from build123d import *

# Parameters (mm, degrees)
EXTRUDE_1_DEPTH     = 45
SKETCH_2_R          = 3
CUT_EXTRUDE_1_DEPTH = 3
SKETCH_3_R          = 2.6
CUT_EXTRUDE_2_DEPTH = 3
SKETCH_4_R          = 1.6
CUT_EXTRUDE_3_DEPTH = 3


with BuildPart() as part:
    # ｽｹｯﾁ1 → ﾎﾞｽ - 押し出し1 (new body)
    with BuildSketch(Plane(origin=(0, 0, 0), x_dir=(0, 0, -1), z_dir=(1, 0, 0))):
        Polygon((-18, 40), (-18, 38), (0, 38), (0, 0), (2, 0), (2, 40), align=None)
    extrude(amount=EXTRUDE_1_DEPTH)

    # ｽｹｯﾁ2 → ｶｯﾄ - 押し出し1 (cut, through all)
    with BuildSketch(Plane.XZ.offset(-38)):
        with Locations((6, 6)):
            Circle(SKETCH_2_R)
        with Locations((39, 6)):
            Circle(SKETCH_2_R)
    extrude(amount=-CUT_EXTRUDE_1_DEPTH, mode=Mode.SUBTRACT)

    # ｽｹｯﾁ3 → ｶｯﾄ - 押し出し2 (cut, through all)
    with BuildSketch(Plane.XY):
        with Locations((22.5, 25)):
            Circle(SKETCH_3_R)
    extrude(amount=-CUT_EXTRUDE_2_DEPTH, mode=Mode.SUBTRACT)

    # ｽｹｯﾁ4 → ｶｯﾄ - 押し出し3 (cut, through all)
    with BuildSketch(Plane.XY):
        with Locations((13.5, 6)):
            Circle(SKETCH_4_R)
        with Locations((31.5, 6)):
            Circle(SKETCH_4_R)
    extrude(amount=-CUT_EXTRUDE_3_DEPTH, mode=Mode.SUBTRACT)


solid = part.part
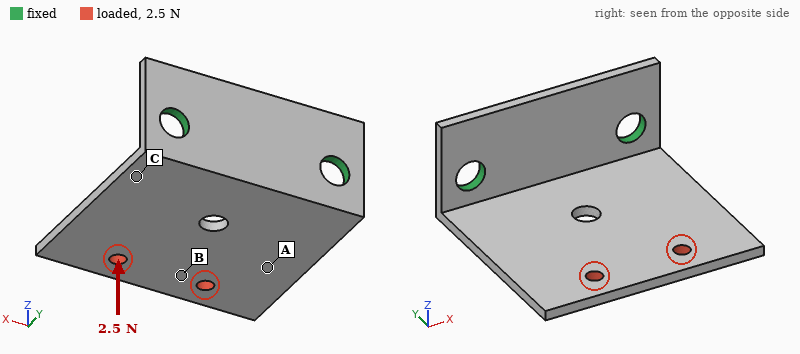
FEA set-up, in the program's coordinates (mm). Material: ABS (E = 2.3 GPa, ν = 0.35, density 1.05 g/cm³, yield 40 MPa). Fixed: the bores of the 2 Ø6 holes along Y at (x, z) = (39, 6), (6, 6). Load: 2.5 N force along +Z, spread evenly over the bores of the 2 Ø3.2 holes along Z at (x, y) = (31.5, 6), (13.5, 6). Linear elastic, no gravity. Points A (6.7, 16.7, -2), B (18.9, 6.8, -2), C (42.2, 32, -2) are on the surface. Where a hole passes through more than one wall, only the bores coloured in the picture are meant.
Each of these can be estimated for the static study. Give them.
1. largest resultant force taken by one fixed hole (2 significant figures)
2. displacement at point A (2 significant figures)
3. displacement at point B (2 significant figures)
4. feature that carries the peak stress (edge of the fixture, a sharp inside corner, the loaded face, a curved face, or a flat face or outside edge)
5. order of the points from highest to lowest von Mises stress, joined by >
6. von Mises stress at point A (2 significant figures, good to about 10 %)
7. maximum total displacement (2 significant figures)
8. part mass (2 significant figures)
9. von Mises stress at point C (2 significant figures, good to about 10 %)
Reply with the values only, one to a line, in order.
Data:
1.3 N
0.34 mm
0.59 mm
a flat face or outside edge
C > A > B
0.96 MPa
0.76 mm
5.3 g
2.2 MPa
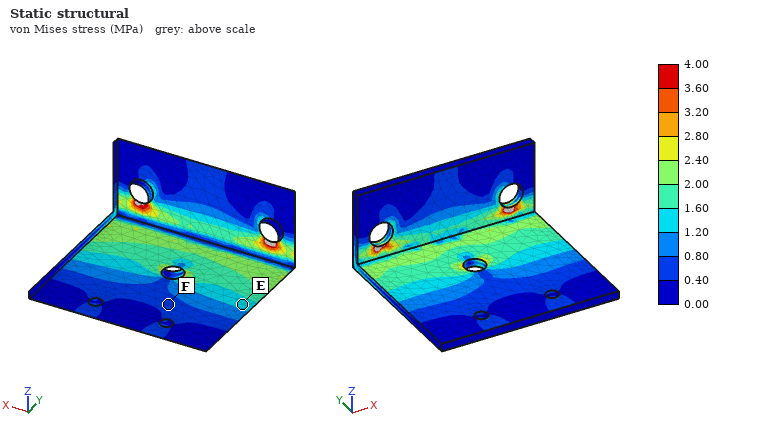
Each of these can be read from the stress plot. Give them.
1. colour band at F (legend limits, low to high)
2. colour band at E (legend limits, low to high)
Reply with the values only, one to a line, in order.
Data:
0.40 to 0.80 MPa
1.20 to 1.60 MPa
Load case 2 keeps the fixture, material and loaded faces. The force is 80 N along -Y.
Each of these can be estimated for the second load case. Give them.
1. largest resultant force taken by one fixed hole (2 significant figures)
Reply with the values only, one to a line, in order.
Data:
41 N
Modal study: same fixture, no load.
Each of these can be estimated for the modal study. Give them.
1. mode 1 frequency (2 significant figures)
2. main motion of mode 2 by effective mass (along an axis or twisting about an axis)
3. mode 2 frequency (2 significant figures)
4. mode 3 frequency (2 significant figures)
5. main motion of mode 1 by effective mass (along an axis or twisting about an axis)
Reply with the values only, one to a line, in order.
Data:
270 Hz
twisting about Y
630 Hz
1600 Hz
along Z
